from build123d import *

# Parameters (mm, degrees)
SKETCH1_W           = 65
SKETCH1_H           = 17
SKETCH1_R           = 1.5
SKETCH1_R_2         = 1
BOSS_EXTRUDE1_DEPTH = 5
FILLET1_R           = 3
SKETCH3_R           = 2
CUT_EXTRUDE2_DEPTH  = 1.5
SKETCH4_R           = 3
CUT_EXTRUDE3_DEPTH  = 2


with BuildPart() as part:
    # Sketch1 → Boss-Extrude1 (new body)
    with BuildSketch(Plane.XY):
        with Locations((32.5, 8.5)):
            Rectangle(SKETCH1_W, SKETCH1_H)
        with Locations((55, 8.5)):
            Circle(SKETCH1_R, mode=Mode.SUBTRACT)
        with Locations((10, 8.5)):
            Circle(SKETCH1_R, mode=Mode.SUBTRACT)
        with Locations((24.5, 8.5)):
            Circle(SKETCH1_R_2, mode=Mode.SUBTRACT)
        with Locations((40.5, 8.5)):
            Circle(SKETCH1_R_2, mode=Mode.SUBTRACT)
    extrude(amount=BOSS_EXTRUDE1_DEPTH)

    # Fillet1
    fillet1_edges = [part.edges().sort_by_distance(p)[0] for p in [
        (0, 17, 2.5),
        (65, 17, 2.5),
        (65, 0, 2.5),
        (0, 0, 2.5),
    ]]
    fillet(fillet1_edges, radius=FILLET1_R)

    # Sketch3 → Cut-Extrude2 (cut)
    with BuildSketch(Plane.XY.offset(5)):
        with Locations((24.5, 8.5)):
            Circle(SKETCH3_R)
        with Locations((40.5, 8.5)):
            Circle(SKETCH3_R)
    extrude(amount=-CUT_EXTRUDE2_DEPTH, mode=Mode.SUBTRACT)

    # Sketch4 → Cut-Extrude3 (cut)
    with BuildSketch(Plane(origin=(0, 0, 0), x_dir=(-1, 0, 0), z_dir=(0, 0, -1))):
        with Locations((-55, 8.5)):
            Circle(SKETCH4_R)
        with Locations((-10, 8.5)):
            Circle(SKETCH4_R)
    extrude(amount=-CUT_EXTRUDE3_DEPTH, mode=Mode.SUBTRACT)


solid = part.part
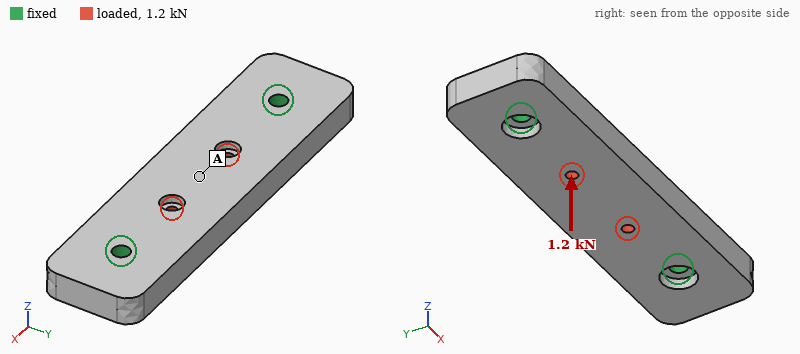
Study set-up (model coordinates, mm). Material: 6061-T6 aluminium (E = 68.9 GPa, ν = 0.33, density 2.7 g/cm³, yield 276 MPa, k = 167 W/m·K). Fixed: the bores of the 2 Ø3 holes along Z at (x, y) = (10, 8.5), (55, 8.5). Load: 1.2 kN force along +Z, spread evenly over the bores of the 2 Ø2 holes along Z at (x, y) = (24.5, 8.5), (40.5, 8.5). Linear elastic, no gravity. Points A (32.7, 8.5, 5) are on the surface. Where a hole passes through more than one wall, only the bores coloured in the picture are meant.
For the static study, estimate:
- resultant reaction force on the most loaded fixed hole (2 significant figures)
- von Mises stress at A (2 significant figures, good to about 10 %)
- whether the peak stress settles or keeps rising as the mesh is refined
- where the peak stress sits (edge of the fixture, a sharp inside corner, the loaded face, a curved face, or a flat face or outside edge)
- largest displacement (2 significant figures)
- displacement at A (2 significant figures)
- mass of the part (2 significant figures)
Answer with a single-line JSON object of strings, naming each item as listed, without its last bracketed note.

{"resultant reaction force on the most loaded fixed hole": "850 N", "von Mises stress at A": "38 MPa", "whether the peak stress settles or keeps rising as the mesh is refined": "keeps rising", "where the peak stress sits": "edge of the fixture", "largest displacement": "63 µm", "displacement at A": "61 µm", "mass of the part": "14 g"}
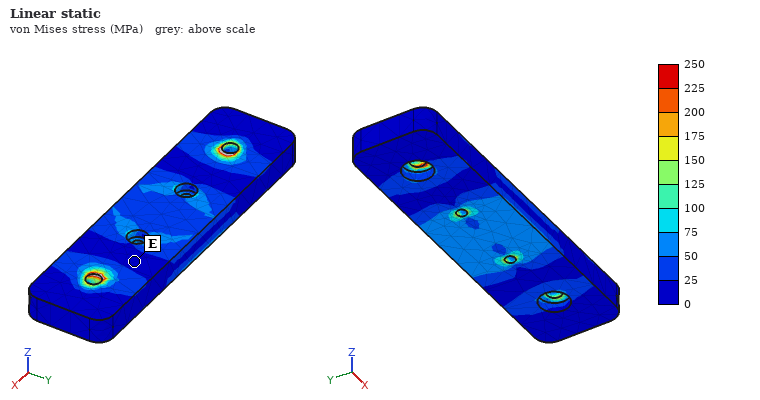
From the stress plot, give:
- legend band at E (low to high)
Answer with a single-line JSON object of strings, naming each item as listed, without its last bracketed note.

{"legend band at E": "0 to 25 MPa"}
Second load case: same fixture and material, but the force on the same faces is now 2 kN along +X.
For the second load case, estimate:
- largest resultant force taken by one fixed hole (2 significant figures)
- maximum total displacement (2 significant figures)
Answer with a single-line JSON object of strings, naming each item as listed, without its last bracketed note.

{"largest resultant force taken by one fixed hole": "1.0 kN", "maximum total displacement": "5.9 µm"}
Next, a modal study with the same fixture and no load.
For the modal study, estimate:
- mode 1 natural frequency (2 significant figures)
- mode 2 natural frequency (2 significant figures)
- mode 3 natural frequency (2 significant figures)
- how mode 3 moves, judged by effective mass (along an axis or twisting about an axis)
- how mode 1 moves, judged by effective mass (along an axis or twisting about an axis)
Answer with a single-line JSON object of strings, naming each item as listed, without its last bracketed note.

{"mode 1 natural frequency": "9000 Hz", "mode 2 natural frequency": "13 kHz", "mode 3 natural frequency": "17 kHz", "how mode 3 moves, judged by effective mass": "along Y", "how mode 1 moves, judged by effective mass": "along Z"}
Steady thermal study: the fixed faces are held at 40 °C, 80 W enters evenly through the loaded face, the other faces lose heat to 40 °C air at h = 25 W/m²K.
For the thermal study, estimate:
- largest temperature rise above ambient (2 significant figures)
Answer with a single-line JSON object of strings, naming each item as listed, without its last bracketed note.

{"largest temperature rise above ambient": "65 K"}
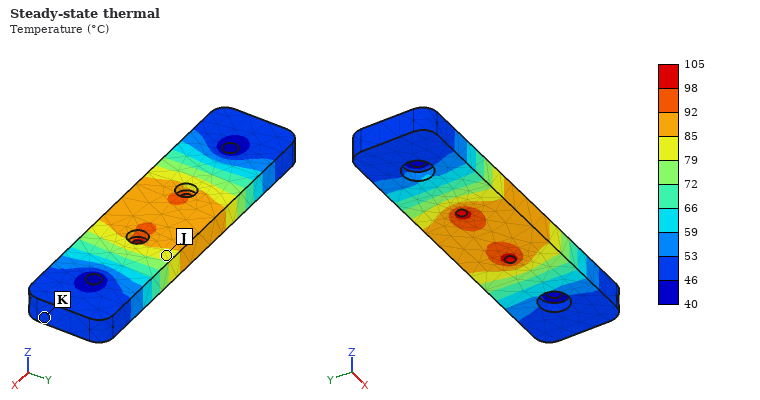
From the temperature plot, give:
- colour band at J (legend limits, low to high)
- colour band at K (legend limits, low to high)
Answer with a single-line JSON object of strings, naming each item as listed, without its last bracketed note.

{"colour band at J": "79 to 85 °C", "colour band at K": "46 to 53 °C"}
